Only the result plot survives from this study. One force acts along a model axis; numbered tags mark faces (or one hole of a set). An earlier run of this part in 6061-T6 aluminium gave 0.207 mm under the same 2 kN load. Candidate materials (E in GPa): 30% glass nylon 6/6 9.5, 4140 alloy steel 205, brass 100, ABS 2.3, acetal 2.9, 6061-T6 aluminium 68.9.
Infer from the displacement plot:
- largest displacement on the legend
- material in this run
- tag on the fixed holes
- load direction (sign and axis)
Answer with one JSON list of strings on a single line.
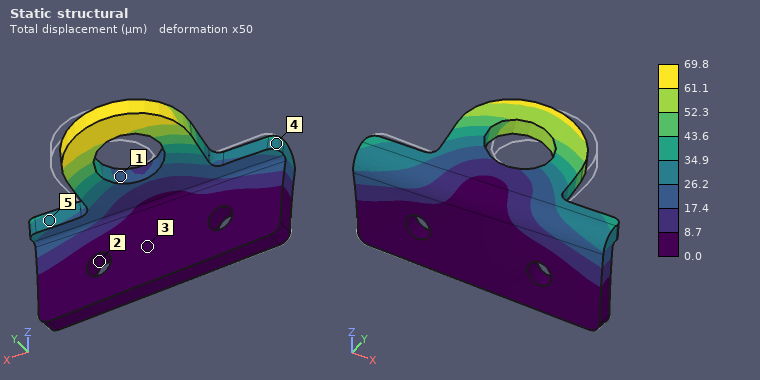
["69.8 µm", "4140 alloy steel", "2", "-X"]
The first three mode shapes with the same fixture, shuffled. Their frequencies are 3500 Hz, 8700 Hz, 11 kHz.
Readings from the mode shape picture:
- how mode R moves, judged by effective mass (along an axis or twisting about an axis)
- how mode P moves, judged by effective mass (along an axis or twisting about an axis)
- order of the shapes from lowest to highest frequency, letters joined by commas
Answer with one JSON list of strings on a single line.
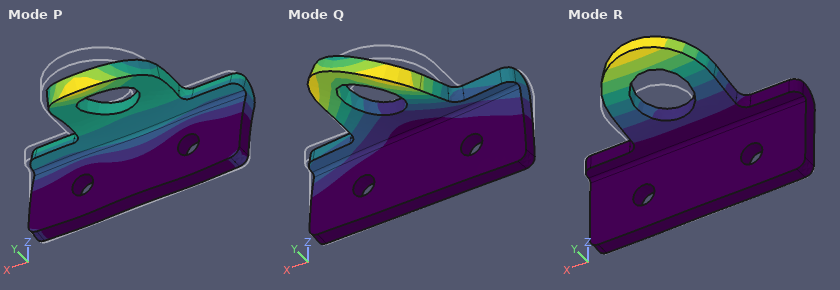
["along Z", "along Y", "R, Q, P"]
